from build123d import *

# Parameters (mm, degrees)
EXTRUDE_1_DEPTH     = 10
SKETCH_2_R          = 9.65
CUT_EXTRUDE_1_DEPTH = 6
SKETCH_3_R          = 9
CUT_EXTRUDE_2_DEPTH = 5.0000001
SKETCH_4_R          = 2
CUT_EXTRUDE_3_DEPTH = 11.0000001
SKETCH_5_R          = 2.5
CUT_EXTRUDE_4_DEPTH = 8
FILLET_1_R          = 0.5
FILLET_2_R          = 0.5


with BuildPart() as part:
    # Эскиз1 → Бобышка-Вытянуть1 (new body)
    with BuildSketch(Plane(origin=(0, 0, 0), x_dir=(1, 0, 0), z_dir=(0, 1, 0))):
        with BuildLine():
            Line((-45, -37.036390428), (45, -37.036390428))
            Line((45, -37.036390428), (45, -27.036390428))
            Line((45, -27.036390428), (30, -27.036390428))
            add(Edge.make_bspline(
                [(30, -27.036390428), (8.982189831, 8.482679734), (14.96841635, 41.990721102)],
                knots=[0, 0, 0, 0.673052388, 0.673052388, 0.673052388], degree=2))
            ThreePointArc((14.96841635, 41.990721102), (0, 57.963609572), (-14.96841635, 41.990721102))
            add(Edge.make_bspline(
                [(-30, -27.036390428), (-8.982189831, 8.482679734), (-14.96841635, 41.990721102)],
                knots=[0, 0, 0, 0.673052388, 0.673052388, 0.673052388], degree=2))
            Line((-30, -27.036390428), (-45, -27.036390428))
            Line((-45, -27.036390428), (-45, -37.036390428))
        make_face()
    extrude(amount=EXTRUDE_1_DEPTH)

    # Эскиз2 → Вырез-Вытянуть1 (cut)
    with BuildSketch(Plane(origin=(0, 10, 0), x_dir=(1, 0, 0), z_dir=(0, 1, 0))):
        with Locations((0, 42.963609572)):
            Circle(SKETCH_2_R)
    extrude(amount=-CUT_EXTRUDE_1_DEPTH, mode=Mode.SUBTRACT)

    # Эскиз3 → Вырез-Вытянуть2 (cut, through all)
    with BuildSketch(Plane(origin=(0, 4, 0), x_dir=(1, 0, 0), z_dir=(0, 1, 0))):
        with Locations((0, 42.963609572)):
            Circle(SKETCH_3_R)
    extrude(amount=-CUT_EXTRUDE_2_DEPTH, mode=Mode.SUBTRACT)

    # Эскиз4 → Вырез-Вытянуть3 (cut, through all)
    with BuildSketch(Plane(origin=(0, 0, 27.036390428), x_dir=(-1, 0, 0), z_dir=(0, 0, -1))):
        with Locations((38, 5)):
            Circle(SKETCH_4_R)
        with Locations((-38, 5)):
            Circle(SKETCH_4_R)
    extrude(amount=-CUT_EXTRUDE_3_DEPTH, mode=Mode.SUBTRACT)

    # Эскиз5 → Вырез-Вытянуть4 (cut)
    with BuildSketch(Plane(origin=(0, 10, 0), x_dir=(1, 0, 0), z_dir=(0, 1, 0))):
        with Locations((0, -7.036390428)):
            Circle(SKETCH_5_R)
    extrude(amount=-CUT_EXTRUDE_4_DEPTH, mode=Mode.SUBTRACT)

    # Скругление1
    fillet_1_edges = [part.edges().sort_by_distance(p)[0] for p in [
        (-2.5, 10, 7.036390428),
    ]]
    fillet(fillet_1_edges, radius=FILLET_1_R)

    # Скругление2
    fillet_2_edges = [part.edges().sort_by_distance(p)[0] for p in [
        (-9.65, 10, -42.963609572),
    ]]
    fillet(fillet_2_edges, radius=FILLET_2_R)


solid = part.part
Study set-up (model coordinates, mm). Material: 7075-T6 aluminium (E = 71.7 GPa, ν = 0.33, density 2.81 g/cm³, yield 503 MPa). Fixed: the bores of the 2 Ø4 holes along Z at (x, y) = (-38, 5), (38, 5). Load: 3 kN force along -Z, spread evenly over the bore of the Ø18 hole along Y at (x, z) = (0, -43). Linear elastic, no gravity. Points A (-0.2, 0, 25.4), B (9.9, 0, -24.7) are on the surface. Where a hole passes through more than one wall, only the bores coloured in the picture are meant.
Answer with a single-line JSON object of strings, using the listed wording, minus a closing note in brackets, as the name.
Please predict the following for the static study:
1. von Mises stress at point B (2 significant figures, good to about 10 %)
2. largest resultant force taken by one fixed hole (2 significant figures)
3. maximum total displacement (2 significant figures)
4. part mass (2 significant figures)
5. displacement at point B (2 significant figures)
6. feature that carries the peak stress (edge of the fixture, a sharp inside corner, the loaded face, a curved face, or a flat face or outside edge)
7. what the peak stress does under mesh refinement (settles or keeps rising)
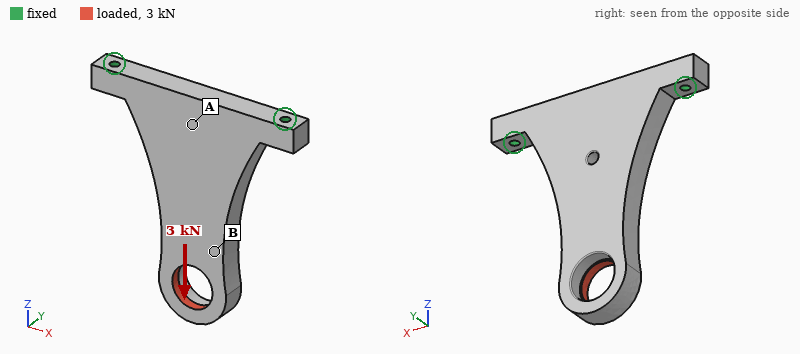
{"von Mises stress at point B": "34 MPa", "largest resultant force taken by one fixed hole": "1.8 kN", "maximum total displacement": "0.31 mm", "part mass": "97 g", "displacement at point B": "0.15 mm", "feature that carries the peak stress": "edge of the fixture", "what the peak stress does under mesh refinement": "keeps rising"}
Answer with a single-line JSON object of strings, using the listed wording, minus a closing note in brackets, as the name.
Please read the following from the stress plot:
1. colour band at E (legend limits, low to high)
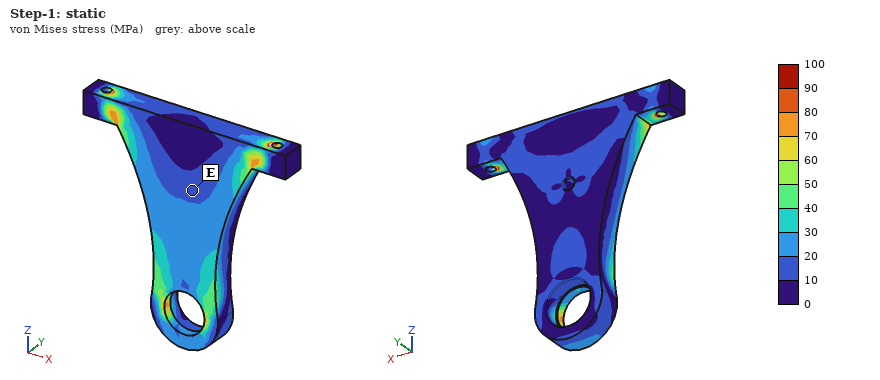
{"colour band at E": "10 to 20 MPa"}
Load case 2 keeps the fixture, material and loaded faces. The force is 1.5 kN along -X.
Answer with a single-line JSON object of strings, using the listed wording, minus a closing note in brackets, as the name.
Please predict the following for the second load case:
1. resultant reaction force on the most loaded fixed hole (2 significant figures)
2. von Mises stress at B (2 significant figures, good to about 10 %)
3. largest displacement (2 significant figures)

{"resultant reaction force on the most loaded fixed hole": "1.9 kN", "von Mises stress at B": "19 MPa", "largest displacement": "0.15 mm"}
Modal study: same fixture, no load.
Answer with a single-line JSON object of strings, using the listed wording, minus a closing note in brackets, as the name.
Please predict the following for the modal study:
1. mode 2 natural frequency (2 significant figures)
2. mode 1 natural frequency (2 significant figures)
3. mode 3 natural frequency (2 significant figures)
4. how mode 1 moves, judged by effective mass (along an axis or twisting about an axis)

{"mode 2 natural frequency": "4400 Hz", "mode 1 natural frequency": "860 Hz", "mode 3 natural frequency": "4500 Hz", "how mode 1 moves, judged by effective mass": "along Y"}
